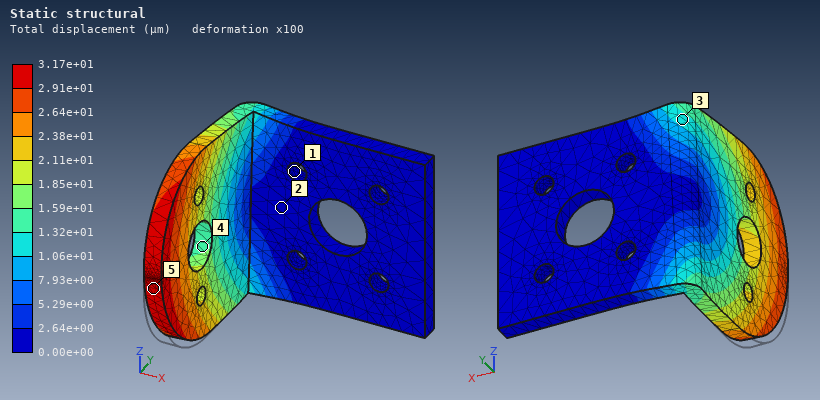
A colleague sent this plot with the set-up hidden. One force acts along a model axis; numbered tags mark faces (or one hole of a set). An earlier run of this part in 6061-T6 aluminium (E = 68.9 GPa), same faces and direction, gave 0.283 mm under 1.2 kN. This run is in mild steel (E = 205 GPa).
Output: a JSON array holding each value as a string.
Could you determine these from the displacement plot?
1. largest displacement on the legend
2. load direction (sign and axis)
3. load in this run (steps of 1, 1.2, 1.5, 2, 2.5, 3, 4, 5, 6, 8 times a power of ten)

["3.17e+01 µm", "+Z", "400 N"]
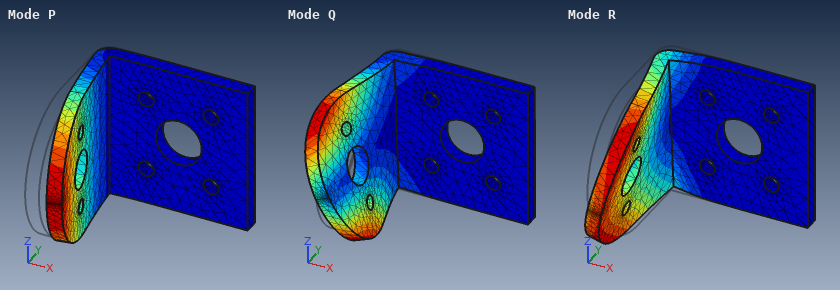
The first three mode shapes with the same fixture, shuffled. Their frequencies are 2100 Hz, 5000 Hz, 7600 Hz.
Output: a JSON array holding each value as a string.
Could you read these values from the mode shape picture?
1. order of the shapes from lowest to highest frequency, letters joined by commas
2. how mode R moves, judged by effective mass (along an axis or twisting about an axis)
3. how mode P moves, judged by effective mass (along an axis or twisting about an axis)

["P, R, Q", "along Z", "along X"]
